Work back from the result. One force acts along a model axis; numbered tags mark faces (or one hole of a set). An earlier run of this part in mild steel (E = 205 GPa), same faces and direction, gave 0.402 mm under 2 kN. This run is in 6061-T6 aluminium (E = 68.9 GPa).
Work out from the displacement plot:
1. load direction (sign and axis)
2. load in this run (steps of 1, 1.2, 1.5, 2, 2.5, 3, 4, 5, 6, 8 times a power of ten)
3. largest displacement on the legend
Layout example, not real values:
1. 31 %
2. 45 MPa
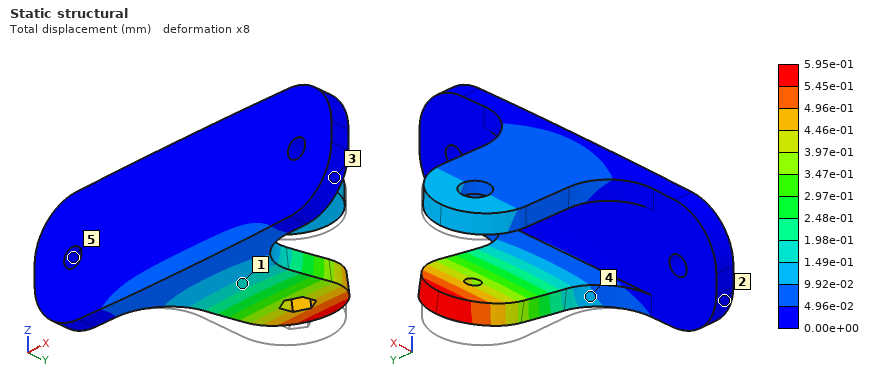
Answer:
1. +Z
2. 1 kN
3. 5.95e-01 mm
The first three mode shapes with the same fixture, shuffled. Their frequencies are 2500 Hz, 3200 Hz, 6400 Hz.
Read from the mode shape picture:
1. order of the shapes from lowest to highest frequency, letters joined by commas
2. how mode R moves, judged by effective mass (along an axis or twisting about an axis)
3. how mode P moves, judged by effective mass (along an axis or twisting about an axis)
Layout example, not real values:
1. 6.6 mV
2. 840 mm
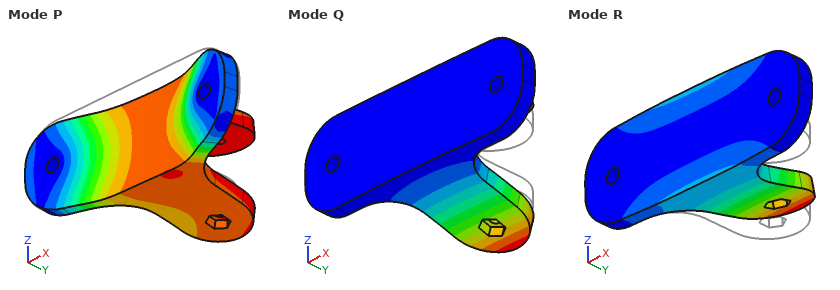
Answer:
1. R, Q, P
2. along Z
3. along Y
